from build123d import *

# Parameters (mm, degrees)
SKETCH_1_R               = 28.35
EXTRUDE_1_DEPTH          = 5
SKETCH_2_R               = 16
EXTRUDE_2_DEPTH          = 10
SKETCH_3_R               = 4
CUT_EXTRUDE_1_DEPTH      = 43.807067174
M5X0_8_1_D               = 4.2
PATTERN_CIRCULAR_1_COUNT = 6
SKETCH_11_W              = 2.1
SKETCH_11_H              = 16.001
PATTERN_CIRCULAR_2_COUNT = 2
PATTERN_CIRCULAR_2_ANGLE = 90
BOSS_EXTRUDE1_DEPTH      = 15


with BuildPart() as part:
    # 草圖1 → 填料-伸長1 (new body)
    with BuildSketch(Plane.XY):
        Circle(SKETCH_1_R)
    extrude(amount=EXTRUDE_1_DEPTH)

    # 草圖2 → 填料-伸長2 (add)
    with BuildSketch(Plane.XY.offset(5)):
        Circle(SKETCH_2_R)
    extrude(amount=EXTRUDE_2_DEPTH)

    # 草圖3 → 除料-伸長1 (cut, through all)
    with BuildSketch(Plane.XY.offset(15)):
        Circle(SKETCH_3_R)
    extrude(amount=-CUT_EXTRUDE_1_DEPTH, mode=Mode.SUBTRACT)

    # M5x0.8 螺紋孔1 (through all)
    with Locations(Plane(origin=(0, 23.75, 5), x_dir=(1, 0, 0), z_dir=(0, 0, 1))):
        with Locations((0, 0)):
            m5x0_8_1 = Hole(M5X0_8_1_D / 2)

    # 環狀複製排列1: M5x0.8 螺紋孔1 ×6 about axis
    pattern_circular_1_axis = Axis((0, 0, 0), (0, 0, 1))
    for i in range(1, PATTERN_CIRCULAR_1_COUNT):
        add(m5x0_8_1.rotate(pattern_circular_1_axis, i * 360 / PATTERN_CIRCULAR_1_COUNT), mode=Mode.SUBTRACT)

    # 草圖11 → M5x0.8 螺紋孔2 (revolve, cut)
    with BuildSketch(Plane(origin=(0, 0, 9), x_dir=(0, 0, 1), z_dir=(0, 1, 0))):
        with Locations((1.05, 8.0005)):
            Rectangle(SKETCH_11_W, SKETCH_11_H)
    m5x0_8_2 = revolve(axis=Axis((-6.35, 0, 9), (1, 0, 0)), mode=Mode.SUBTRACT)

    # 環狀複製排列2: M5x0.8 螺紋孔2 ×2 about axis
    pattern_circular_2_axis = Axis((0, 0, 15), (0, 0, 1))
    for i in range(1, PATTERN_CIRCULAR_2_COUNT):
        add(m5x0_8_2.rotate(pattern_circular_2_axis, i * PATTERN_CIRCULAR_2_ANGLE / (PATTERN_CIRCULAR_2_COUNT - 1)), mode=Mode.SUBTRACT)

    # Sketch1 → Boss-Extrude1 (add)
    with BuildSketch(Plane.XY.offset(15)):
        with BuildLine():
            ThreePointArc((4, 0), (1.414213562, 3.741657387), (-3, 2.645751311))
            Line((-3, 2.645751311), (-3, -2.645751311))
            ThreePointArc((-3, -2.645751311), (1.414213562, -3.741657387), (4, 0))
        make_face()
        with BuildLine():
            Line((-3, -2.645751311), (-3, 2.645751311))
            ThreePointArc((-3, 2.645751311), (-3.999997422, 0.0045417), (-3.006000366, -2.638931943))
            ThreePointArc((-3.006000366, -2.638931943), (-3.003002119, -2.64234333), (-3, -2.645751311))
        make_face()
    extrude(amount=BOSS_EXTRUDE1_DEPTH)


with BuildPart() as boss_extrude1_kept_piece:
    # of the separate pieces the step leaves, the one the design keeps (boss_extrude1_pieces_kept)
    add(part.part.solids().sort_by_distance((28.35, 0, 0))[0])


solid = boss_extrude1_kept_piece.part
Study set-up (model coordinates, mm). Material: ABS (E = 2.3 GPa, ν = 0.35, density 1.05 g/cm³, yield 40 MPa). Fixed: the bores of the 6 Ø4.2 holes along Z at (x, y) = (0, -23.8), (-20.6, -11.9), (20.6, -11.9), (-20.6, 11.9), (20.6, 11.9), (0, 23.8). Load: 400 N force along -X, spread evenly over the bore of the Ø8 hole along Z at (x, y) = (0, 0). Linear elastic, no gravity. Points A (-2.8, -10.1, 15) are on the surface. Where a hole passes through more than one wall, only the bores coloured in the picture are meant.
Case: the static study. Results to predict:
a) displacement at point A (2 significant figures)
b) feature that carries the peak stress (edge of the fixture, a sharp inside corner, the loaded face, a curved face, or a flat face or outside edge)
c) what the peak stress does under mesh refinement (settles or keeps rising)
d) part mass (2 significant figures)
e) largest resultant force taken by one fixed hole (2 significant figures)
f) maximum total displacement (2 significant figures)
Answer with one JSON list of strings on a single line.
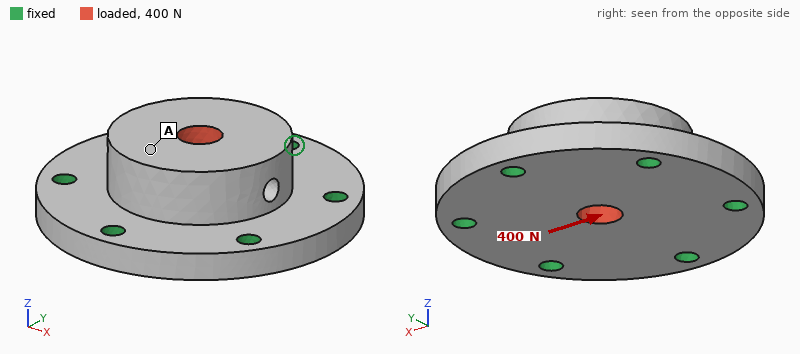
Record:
["15 µm", "edge of the fixture", "keeps rising", "20 g", "94 N", "20 µm"]
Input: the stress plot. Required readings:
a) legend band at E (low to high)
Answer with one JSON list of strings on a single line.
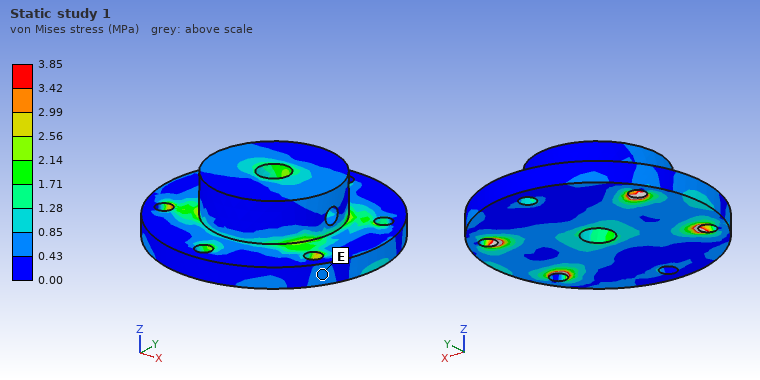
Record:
["0.43 to 0.85 MPa"]
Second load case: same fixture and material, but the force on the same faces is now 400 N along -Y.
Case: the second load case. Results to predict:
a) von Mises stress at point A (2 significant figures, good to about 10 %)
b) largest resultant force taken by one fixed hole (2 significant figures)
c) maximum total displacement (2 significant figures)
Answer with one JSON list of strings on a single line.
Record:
["0.69 MPa", "110 N", "20 µm"]
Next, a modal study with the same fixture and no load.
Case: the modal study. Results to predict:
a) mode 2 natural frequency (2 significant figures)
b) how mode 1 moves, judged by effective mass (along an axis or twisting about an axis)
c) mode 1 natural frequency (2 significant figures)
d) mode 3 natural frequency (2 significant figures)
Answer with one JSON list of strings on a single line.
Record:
["7000 Hz", "along Z", "5400 Hz", "7000 Hz"]
